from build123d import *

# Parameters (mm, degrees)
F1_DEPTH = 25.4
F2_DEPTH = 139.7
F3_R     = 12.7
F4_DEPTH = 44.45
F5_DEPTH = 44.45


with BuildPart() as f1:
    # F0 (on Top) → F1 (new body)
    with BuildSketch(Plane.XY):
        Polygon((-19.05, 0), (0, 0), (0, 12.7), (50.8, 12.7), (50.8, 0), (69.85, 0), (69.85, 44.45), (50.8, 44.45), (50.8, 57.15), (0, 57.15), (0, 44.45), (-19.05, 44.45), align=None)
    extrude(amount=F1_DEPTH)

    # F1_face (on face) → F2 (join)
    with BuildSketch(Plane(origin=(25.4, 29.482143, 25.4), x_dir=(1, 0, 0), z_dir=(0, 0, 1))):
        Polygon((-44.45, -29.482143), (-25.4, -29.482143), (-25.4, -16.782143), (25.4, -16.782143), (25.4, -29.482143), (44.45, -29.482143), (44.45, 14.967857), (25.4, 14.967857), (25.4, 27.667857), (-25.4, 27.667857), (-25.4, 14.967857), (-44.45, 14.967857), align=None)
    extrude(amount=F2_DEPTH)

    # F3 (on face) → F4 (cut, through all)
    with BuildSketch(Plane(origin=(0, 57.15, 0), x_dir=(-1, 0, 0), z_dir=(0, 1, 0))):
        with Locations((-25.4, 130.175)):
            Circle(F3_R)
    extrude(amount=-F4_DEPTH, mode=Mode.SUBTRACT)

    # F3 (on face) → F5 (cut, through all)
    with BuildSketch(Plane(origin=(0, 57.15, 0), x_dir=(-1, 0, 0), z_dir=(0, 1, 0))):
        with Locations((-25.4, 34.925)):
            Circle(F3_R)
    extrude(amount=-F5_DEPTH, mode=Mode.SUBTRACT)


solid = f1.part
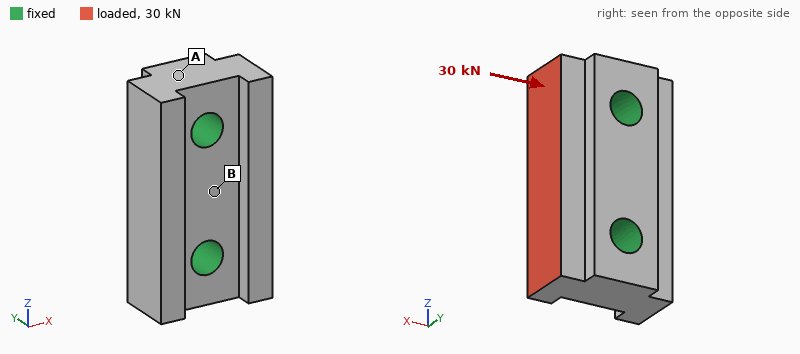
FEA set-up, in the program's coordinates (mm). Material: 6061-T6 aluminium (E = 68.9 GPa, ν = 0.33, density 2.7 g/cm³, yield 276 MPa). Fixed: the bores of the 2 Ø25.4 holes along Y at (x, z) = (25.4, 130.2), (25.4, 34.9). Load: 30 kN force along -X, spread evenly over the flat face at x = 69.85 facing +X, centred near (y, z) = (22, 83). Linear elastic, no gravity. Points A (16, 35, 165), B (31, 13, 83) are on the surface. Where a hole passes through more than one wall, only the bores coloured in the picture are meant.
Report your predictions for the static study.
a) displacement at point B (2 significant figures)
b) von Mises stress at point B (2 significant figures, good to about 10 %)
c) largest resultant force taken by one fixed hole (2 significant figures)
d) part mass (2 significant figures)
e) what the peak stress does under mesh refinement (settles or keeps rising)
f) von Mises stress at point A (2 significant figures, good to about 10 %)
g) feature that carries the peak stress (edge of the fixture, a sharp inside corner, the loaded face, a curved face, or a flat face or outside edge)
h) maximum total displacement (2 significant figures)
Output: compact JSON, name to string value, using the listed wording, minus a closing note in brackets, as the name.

{"displacement at point B": "4.0 µm", "von Mises stress at point B": "5.3 MPa", "largest resultant force taken by one fixed hole": "15 kN", "part mass": "1.6 kg", "what the peak stress does under mesh refinement": "keeps rising", "von Mises stress at point A": "2.3 MPa", "feature that carries the peak stress": "edge of the fixture", "maximum total displacement": "14 µm"}
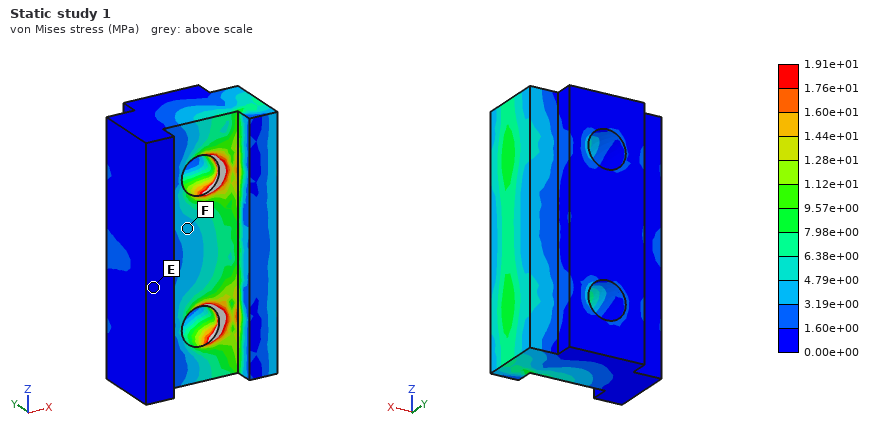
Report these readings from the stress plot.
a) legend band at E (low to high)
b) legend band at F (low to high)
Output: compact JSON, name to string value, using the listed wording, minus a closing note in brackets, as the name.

{"legend band at E": "0.00e+00 to 1.60e+00 MPa", "legend band at F": "3.19e+00 to 4.79e+00 MPa"}
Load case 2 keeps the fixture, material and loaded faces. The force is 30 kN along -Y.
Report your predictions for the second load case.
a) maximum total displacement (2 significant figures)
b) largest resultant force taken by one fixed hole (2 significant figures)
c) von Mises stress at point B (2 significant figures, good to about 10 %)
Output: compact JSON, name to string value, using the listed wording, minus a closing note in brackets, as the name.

{"maximum total displacement": "35 µm", "largest resultant force taken by one fixed hole": "15 kN", "von Mises stress at point B": "11 MPa"}
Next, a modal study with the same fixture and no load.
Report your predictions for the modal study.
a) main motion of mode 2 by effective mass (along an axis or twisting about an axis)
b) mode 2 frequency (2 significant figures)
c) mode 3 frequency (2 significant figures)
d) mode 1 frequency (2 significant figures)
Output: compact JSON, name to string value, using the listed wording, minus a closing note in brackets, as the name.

{"main motion of mode 2 by effective mass": "along Y", "mode 2 frequency": "11 kHz", "mode 3 frequency": "12 kHz", "mode 1 frequency": "9700 Hz"}
